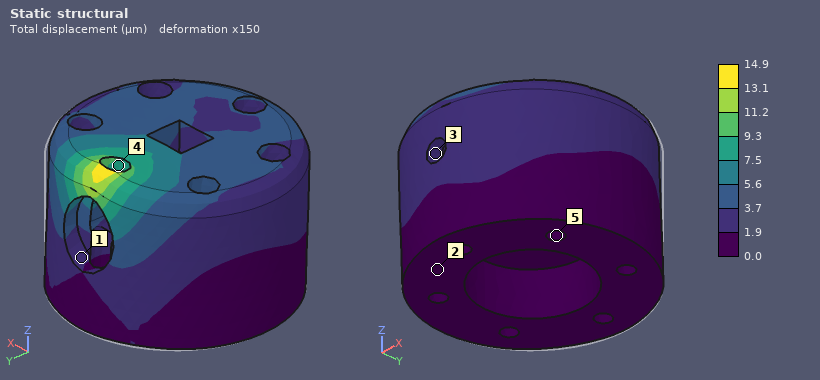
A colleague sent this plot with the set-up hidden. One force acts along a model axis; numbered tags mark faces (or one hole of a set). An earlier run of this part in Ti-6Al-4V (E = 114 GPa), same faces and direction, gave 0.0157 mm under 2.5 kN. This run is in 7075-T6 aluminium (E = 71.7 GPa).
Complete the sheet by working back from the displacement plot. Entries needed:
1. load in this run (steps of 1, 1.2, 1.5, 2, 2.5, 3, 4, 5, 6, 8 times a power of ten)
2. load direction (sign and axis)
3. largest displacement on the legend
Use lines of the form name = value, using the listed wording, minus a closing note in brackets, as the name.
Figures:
load in this run = 1.5 kN
load direction = -Y
largest displacement on the legend = 14.9 µm
